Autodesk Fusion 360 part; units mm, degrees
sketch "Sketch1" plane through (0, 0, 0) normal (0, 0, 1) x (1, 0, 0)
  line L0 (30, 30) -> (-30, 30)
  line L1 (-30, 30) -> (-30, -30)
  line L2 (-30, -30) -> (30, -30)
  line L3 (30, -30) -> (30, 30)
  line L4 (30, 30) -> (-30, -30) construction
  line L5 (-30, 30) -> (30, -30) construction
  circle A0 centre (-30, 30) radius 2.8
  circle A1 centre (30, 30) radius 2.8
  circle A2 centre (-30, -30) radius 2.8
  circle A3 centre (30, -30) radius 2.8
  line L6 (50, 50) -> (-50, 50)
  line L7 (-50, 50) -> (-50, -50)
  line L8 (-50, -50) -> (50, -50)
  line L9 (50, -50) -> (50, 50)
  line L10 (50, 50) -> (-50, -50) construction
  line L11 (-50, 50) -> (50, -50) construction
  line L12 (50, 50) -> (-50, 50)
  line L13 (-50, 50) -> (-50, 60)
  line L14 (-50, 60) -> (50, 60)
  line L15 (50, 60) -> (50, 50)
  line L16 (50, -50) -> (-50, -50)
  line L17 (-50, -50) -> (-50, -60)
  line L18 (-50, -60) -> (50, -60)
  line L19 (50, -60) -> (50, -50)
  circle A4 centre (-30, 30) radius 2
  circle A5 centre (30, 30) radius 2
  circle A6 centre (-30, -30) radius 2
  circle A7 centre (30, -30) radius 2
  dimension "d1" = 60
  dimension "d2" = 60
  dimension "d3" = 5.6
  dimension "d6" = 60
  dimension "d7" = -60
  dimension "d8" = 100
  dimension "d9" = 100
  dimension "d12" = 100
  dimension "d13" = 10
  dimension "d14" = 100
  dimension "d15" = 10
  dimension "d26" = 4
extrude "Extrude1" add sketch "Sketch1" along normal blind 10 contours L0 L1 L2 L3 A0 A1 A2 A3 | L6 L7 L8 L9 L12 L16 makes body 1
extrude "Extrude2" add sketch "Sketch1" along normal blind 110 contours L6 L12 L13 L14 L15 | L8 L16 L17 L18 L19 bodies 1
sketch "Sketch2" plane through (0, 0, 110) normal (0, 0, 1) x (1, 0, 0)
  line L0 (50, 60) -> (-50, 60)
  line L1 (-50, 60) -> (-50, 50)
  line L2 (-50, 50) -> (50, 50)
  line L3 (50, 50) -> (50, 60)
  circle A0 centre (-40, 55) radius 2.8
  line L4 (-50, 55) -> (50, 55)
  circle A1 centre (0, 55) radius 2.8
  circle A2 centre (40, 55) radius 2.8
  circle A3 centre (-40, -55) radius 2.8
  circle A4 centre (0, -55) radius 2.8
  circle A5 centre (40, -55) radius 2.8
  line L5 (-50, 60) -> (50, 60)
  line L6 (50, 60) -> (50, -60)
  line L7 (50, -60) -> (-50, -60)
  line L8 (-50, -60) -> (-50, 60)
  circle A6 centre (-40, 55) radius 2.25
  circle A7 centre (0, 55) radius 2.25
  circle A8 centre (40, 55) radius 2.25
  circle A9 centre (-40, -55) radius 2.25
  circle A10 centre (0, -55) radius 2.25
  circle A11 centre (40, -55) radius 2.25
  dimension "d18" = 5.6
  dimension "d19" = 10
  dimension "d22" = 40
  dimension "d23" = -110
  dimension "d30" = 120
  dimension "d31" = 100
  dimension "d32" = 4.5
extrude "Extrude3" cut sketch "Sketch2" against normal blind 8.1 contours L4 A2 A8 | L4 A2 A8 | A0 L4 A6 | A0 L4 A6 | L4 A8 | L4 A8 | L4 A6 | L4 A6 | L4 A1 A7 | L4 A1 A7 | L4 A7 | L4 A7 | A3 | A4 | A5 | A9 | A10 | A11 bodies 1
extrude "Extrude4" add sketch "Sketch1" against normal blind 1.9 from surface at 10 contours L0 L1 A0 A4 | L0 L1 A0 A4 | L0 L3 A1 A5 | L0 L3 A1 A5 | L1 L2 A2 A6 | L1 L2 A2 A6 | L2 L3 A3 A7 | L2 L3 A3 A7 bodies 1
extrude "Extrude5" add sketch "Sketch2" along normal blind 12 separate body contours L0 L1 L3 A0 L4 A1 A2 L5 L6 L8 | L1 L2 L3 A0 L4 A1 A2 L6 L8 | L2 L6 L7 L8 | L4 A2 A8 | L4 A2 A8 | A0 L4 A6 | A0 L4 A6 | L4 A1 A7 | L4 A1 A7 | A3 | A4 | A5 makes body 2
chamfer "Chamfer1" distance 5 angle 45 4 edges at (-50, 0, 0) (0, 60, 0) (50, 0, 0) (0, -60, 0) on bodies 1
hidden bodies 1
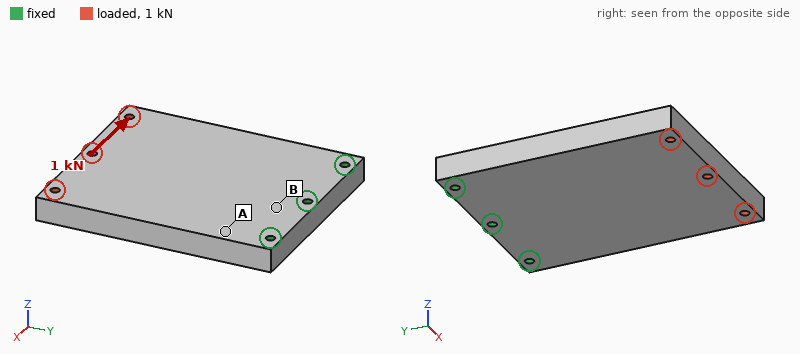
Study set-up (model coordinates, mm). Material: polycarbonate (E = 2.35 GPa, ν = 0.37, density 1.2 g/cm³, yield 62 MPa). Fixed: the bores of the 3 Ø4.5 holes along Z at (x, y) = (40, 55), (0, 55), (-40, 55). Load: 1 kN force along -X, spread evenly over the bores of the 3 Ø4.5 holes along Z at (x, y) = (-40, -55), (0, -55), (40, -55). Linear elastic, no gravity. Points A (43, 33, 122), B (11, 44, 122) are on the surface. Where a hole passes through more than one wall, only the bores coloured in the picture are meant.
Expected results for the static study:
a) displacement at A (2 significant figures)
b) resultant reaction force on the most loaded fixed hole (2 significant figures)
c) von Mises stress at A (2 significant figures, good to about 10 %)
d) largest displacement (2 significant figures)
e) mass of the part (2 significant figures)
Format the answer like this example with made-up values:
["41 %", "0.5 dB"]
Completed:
["0.079 mm", "1.4 kN", "4.2 MPa", "0.43 mm", "170 g"]
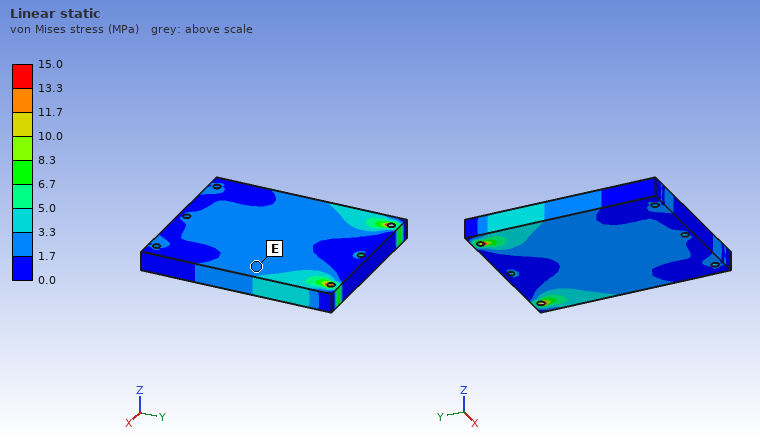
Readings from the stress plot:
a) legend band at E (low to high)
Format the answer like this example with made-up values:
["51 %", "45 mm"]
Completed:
["1.7 to 3.3 MPa"]
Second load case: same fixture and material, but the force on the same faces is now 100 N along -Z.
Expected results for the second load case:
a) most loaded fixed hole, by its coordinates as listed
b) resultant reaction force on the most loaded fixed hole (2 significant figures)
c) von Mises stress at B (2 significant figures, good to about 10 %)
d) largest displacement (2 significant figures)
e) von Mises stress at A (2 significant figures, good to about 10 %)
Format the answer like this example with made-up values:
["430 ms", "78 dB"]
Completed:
["(0, 55)", "80 N", "3.2 MPa", "1.7 mm", "3.9 MPa"]
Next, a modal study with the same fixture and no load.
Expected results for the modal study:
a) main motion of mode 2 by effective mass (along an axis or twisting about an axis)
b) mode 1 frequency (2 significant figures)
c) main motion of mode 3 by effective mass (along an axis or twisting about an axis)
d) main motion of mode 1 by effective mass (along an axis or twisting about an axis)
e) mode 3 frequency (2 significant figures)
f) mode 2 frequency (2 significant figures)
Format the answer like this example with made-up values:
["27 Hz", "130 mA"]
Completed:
["twisting about Y", "190 Hz", "along X", "along Z", "1100 Hz", "520 Hz"]
